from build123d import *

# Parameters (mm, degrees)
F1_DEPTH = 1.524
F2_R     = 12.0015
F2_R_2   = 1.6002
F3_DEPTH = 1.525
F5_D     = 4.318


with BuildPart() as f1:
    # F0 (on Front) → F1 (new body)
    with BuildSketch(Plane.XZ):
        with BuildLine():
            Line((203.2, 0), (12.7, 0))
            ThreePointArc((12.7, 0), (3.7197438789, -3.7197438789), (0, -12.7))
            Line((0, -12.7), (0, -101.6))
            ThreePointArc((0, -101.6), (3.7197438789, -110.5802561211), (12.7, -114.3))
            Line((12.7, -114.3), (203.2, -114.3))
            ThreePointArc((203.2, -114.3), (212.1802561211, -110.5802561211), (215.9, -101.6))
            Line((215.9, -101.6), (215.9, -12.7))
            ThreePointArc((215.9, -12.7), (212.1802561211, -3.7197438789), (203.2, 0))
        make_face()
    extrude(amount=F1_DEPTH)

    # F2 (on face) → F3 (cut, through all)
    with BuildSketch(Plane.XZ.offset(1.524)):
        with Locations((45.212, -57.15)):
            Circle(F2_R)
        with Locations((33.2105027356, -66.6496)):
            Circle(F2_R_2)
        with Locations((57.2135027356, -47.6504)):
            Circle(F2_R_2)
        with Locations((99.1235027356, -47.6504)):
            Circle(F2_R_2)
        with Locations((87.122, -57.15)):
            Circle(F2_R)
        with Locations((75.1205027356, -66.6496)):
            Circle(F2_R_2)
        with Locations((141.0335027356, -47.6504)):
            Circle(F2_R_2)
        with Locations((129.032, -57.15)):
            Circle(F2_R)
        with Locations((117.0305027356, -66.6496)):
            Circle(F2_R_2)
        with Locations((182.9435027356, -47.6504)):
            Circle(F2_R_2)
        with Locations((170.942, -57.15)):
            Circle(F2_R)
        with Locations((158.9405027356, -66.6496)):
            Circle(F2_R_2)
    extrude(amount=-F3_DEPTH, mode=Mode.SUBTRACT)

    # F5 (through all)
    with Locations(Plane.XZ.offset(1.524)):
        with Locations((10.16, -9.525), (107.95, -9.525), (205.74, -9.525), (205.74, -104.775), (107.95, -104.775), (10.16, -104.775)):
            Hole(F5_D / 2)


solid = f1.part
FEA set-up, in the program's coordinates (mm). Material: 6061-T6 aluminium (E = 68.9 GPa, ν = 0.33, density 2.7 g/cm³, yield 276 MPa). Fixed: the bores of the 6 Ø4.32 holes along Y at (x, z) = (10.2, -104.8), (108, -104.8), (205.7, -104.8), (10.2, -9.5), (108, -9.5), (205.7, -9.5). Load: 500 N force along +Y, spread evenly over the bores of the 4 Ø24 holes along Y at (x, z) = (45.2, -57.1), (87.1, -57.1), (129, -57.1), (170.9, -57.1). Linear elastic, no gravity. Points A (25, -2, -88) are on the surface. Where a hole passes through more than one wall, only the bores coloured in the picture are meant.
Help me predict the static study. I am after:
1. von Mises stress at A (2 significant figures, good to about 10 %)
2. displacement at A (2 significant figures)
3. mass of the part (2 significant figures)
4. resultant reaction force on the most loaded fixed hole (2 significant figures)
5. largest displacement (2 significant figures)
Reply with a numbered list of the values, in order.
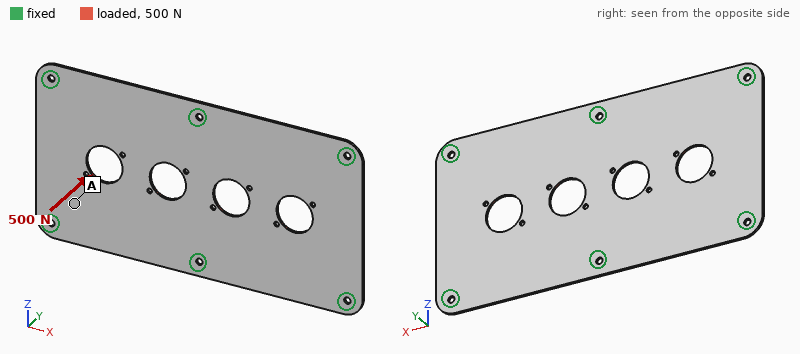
1. 28 MPa
2. 0.40 mm
3. 93 g
4. 160 N
5. 1.5 mm
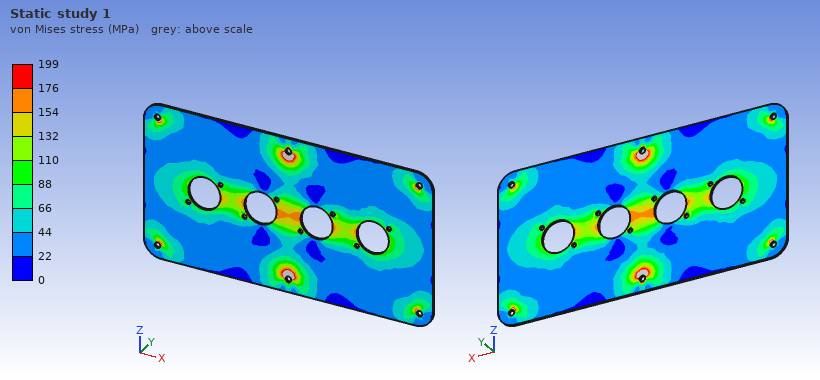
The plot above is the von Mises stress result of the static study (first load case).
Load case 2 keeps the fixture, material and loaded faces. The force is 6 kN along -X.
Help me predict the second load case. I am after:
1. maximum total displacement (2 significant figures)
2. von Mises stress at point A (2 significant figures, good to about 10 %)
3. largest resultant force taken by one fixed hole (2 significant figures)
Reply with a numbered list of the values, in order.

1. 28 µm
2. 19 MPa
3. 1.4 kN
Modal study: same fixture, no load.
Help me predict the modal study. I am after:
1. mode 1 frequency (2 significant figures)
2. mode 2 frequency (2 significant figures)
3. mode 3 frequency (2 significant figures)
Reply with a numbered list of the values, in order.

1. 580 Hz
2. 580 Hz
3. 910 Hz
